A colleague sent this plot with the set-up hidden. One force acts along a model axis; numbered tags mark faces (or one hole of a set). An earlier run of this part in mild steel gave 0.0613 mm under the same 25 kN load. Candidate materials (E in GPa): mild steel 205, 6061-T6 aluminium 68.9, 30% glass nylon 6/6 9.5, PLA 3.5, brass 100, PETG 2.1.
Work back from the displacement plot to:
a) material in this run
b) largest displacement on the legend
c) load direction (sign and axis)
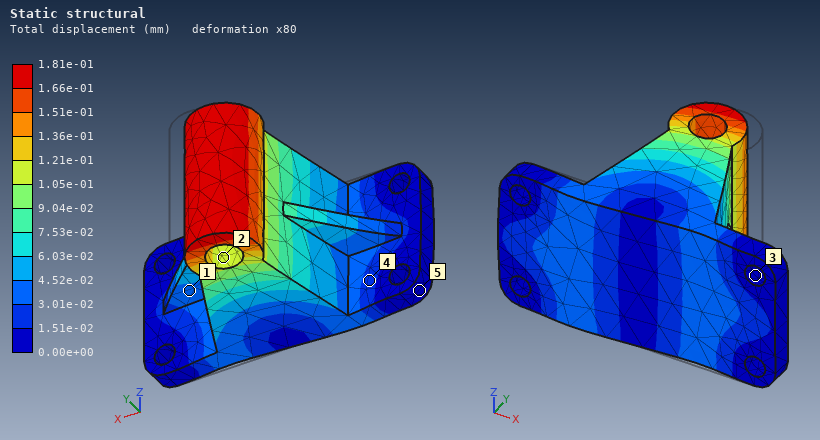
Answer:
6061-T6 aluminium
1.81e-01 mm
-X
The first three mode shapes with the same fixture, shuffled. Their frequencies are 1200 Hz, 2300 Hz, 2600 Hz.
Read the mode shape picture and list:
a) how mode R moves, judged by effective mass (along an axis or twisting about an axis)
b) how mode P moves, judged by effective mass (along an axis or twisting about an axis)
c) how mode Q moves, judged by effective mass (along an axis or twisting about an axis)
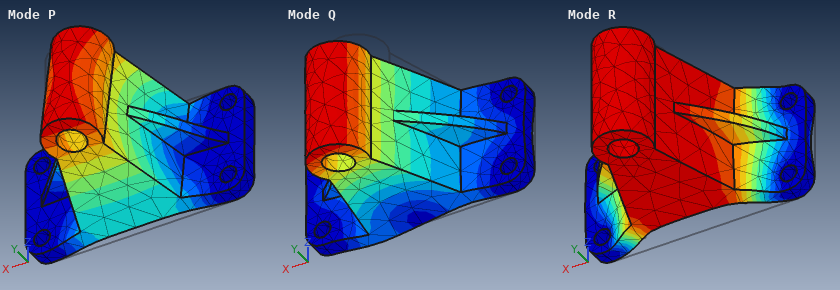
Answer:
along Y
along Z
along X
